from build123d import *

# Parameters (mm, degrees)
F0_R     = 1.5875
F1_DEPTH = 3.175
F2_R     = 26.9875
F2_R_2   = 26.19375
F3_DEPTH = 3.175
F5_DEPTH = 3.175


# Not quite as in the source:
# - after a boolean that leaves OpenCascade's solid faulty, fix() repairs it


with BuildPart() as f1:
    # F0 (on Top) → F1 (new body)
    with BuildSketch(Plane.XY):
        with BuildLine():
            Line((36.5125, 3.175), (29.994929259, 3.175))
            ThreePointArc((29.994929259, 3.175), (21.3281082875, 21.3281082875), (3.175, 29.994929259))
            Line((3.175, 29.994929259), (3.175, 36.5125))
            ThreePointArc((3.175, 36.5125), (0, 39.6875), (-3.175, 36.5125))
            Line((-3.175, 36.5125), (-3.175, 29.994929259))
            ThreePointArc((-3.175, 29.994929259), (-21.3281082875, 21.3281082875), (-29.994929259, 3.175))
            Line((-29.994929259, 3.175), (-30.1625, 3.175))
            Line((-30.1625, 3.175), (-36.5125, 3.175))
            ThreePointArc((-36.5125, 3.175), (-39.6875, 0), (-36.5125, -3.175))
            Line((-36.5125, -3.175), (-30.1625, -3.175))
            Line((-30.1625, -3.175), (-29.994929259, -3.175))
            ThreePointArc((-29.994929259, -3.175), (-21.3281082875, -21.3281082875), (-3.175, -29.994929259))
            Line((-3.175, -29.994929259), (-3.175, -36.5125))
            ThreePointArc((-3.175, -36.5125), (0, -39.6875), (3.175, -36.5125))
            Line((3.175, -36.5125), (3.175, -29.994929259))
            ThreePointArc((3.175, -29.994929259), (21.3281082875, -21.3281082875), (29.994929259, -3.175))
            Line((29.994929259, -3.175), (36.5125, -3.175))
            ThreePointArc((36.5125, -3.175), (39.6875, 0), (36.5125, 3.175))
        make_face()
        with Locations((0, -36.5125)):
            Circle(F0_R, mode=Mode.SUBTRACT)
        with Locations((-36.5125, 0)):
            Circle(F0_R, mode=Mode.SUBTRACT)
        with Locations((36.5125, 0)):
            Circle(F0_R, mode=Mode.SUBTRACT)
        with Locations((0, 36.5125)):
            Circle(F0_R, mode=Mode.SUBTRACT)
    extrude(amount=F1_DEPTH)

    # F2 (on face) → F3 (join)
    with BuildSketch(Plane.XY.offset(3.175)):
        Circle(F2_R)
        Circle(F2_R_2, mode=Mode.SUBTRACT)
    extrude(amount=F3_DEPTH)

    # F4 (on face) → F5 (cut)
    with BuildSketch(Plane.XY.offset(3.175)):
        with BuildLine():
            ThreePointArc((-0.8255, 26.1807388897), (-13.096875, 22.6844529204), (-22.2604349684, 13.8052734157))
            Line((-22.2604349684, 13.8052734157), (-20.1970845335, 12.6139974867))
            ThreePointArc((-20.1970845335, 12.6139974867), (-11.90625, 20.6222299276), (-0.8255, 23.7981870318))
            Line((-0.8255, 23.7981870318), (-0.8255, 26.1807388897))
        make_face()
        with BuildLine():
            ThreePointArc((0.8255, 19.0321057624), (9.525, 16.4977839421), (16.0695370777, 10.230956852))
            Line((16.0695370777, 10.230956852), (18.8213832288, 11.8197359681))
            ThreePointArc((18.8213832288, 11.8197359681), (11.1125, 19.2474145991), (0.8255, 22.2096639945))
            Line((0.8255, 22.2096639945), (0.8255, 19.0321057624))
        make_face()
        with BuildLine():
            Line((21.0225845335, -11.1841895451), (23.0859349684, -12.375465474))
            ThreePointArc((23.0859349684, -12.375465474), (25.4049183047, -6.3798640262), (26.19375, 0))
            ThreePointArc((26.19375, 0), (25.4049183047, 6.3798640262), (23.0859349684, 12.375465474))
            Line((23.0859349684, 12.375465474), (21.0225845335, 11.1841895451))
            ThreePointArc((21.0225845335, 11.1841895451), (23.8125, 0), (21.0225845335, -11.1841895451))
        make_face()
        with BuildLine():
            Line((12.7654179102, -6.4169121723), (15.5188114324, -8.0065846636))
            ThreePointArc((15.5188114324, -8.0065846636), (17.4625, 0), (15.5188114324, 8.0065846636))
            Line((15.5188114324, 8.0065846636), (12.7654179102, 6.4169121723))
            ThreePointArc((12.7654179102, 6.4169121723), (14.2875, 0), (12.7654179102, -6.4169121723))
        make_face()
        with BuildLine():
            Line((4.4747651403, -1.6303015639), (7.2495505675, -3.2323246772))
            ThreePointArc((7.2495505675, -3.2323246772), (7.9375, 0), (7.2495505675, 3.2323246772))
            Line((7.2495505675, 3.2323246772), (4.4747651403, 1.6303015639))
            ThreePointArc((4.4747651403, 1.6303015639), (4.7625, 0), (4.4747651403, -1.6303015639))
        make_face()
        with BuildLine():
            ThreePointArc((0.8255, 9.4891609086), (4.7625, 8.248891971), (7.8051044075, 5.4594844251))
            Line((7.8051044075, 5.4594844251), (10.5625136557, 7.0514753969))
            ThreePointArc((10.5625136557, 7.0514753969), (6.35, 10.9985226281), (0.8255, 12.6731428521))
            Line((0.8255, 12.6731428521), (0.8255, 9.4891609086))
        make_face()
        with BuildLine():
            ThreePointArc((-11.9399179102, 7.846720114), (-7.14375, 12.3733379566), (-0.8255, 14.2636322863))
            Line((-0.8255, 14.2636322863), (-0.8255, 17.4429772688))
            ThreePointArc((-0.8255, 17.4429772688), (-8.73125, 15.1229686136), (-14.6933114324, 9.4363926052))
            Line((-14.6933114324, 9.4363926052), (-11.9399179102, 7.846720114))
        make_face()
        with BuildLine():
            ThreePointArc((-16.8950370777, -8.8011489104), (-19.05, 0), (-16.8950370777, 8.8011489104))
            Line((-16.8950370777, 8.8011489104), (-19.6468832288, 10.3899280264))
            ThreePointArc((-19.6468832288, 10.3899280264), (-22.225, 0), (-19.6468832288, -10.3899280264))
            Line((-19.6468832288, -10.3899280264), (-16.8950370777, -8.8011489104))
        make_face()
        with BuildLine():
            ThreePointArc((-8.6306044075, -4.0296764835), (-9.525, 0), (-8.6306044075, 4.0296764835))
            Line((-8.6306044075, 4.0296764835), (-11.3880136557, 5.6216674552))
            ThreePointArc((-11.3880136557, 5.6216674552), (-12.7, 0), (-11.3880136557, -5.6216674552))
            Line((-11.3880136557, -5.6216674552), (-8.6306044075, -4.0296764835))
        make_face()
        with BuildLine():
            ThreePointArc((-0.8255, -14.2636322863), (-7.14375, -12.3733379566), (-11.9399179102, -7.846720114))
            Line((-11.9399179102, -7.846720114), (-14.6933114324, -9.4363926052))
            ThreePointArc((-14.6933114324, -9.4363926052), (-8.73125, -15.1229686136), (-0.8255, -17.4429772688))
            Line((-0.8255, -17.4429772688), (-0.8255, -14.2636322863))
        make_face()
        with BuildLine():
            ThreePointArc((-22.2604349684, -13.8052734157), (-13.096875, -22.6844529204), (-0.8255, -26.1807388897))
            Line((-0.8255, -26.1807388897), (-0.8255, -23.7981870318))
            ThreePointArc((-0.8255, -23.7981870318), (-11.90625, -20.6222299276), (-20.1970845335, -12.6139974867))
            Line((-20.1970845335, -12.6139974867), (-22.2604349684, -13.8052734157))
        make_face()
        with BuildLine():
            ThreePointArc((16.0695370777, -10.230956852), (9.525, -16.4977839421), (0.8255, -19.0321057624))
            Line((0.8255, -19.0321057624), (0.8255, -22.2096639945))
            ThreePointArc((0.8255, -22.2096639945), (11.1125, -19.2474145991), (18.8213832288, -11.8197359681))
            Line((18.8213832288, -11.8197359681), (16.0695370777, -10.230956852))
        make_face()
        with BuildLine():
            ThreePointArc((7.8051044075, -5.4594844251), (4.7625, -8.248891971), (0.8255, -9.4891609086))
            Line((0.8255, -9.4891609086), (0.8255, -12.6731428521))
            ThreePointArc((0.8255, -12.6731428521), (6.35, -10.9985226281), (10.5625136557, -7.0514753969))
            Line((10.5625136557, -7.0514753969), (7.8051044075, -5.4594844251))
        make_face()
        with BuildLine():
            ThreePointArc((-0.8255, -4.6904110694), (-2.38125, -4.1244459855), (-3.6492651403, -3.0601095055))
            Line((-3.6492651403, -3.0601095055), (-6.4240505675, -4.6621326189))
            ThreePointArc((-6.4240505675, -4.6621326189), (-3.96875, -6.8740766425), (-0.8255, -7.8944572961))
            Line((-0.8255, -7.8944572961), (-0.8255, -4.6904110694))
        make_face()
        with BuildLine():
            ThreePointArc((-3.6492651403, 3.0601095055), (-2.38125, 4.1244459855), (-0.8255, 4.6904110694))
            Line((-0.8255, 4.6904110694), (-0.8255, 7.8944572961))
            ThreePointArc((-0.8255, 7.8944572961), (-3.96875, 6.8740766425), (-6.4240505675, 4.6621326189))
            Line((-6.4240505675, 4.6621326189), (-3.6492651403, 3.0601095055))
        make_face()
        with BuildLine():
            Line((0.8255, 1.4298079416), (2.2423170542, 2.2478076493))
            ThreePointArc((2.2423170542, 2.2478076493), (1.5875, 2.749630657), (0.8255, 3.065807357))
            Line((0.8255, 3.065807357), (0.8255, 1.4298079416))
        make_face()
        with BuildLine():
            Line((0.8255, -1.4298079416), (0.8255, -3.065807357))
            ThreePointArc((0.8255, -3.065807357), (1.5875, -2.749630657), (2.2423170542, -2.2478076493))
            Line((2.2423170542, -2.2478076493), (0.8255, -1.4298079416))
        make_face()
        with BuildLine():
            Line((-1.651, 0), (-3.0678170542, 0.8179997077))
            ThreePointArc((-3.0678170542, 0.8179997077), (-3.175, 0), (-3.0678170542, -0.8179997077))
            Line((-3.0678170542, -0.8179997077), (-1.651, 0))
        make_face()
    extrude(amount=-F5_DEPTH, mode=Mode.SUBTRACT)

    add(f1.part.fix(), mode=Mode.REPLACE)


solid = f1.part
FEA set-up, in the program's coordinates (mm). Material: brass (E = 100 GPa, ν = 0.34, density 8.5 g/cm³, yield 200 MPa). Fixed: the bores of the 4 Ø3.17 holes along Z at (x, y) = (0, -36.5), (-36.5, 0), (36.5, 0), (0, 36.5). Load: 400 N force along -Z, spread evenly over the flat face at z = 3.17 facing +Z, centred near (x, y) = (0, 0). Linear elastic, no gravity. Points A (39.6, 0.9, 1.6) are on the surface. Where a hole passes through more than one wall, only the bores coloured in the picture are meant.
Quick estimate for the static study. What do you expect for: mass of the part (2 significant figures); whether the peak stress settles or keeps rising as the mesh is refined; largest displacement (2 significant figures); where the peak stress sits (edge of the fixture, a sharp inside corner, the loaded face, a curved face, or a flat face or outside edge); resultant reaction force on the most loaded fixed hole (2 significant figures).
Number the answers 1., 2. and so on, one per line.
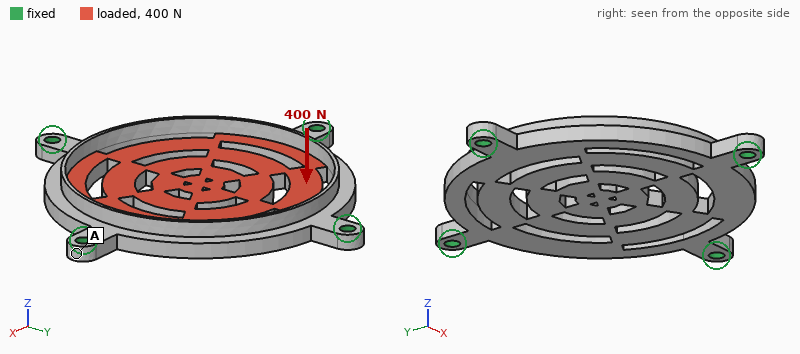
1. 68 g
2. keeps rising
3. 53 µm
4. edge of the fixture
5. 110 N
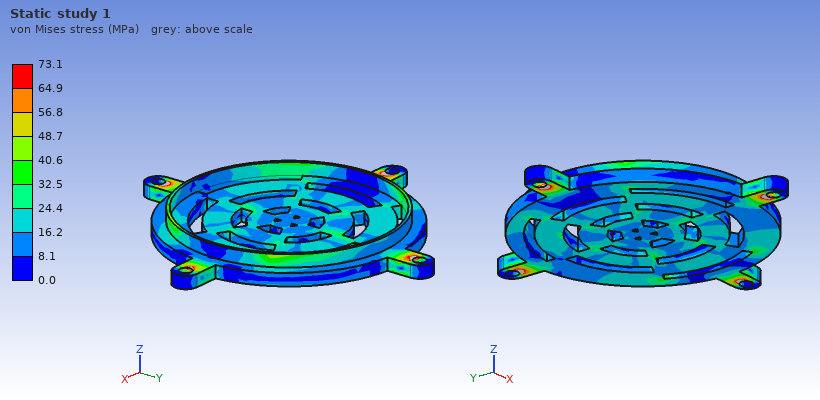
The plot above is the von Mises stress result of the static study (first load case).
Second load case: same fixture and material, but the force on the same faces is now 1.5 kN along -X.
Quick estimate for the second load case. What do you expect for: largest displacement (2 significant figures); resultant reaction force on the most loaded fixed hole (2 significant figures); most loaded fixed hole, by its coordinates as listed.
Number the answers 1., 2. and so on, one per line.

1. 18 µm
2. 660 N
3. (-36.5, 0)
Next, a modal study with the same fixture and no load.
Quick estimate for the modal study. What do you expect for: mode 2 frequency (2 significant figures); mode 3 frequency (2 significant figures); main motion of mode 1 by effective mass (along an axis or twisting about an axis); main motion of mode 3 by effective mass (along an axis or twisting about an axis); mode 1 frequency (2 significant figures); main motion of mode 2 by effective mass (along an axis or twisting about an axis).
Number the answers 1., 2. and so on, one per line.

1. 3600 Hz
2. 3800 Hz
3. along Z
4. twisting about X
5. 2400 Hz
6. twisting about Y
